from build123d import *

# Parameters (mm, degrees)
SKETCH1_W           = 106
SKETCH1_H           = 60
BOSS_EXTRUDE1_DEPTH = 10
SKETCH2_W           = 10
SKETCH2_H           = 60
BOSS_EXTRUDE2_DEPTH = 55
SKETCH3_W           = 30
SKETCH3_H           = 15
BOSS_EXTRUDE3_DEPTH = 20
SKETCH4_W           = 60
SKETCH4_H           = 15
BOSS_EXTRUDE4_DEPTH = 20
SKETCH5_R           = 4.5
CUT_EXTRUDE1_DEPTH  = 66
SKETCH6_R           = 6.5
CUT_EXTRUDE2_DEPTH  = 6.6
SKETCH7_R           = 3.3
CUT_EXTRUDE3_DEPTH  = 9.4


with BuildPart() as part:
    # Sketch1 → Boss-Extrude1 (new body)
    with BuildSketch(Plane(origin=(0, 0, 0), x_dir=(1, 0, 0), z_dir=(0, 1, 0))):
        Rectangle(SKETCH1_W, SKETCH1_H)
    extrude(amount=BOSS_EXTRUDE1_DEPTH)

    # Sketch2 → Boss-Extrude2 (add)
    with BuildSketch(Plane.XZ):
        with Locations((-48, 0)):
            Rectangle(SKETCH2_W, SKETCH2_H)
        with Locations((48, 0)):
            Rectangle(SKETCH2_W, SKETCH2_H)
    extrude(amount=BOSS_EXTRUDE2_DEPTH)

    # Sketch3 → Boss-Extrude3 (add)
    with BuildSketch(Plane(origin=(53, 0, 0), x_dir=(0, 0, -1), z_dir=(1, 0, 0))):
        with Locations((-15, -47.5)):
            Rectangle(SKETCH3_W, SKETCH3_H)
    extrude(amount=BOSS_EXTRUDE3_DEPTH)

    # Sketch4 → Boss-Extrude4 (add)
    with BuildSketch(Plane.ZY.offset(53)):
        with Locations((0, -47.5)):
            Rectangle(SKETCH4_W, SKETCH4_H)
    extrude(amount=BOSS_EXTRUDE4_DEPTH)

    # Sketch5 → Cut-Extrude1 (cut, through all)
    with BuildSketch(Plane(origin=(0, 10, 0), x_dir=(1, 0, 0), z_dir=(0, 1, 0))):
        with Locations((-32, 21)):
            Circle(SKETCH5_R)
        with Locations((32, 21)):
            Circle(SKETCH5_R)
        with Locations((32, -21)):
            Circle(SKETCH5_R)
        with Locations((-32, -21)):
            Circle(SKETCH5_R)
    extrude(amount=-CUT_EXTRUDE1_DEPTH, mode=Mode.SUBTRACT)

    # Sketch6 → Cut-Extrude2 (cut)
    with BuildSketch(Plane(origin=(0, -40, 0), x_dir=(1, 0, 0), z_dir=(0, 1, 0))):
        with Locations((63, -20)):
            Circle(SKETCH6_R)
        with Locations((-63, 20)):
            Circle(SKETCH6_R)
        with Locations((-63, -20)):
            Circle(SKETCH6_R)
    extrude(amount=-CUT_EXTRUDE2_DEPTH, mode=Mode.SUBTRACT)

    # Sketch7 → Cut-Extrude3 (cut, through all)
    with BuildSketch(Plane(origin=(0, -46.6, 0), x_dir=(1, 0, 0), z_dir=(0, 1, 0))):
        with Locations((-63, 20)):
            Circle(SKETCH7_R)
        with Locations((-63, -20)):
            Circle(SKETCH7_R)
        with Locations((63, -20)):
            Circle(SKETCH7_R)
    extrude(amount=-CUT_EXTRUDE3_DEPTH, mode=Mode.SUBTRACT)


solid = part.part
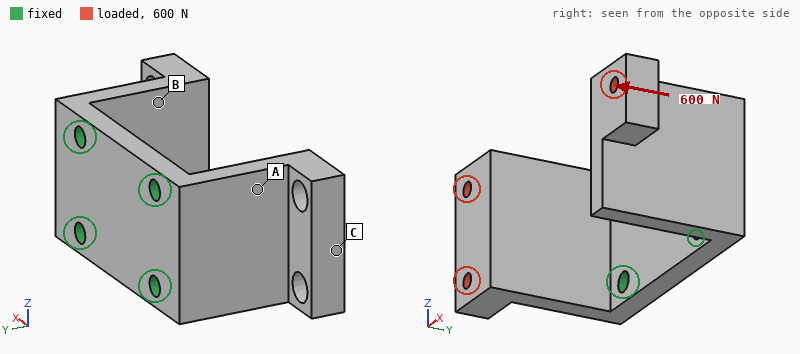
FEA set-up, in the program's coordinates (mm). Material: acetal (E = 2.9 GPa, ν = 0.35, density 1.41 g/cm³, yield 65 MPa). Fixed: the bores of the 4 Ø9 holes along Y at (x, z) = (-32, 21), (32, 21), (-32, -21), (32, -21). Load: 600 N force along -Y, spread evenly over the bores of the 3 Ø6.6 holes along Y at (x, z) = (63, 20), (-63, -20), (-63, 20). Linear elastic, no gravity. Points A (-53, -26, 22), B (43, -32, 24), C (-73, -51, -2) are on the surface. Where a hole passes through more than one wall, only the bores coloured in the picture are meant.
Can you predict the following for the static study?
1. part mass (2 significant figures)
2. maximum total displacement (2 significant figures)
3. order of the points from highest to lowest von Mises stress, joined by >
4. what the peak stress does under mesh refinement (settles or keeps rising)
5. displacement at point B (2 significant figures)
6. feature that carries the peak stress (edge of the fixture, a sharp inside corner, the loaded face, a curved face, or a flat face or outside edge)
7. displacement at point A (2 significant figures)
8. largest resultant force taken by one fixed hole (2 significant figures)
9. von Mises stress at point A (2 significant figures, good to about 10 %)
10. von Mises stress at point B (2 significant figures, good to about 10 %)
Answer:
210 g
1.4 mm
A > B > C
keeps rising
0.30 mm
edge of the fixture
0.46 mm
210 N
6.5 MPa
2.8 MPa
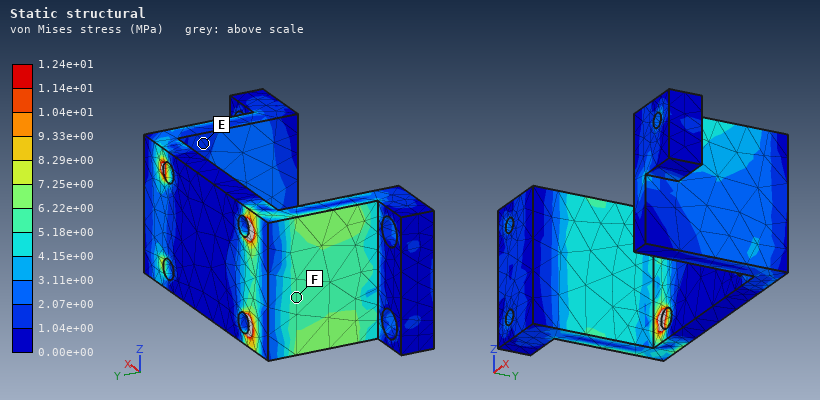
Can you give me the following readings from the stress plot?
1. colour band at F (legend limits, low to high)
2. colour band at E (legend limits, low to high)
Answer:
5.18e+00 to 6.22e+00 MPa
1.04e+00 to 2.07e+00 MPa
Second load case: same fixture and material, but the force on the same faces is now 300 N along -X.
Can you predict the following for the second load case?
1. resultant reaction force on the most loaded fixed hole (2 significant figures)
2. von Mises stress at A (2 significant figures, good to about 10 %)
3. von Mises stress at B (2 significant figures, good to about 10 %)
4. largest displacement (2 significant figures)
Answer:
100 N
4.9 MPa
2.4 MPa
1.6 mm
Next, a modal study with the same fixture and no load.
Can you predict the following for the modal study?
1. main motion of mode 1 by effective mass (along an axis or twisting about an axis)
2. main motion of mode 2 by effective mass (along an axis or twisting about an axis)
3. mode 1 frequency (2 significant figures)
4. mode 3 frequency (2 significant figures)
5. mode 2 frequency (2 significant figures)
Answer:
along X
along X
320 Hz
920 Hz
380 Hz
